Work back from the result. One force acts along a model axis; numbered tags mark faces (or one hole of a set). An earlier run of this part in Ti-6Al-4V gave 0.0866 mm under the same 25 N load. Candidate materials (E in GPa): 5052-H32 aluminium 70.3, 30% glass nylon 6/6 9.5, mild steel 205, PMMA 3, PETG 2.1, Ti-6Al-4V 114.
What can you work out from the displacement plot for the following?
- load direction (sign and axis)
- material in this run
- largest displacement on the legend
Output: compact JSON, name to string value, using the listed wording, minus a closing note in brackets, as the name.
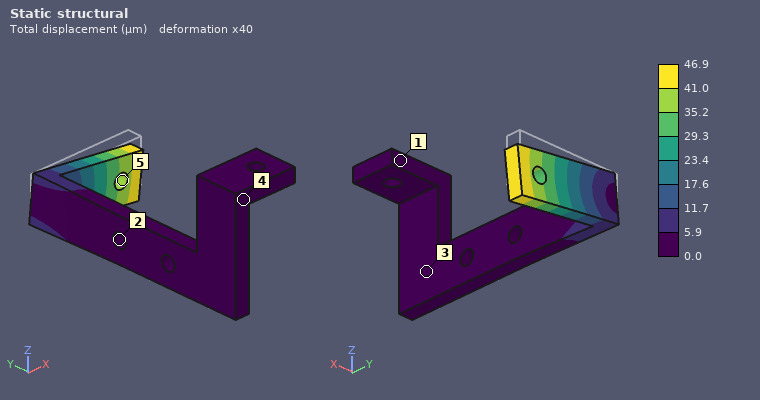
{"load direction": "-Z", "material in this run": "mild steel", "largest displacement on the legend": "46.9 µm"}
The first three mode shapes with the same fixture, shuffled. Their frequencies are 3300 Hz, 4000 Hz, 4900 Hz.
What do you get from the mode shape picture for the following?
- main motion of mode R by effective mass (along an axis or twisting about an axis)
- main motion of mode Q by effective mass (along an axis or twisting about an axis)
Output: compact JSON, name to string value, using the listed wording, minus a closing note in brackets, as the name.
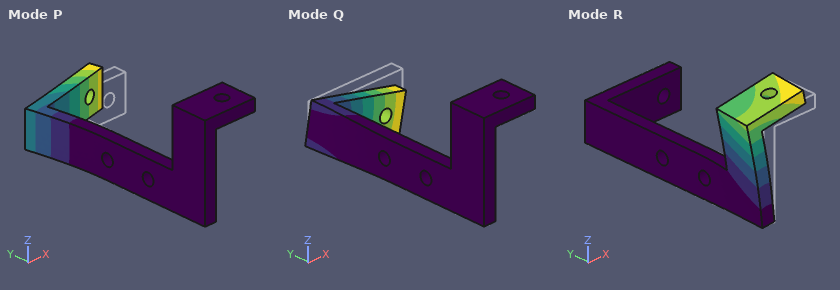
{"main motion of mode R by effective mass": "along X", "main motion of mode Q by effective mass": "along Z"}
